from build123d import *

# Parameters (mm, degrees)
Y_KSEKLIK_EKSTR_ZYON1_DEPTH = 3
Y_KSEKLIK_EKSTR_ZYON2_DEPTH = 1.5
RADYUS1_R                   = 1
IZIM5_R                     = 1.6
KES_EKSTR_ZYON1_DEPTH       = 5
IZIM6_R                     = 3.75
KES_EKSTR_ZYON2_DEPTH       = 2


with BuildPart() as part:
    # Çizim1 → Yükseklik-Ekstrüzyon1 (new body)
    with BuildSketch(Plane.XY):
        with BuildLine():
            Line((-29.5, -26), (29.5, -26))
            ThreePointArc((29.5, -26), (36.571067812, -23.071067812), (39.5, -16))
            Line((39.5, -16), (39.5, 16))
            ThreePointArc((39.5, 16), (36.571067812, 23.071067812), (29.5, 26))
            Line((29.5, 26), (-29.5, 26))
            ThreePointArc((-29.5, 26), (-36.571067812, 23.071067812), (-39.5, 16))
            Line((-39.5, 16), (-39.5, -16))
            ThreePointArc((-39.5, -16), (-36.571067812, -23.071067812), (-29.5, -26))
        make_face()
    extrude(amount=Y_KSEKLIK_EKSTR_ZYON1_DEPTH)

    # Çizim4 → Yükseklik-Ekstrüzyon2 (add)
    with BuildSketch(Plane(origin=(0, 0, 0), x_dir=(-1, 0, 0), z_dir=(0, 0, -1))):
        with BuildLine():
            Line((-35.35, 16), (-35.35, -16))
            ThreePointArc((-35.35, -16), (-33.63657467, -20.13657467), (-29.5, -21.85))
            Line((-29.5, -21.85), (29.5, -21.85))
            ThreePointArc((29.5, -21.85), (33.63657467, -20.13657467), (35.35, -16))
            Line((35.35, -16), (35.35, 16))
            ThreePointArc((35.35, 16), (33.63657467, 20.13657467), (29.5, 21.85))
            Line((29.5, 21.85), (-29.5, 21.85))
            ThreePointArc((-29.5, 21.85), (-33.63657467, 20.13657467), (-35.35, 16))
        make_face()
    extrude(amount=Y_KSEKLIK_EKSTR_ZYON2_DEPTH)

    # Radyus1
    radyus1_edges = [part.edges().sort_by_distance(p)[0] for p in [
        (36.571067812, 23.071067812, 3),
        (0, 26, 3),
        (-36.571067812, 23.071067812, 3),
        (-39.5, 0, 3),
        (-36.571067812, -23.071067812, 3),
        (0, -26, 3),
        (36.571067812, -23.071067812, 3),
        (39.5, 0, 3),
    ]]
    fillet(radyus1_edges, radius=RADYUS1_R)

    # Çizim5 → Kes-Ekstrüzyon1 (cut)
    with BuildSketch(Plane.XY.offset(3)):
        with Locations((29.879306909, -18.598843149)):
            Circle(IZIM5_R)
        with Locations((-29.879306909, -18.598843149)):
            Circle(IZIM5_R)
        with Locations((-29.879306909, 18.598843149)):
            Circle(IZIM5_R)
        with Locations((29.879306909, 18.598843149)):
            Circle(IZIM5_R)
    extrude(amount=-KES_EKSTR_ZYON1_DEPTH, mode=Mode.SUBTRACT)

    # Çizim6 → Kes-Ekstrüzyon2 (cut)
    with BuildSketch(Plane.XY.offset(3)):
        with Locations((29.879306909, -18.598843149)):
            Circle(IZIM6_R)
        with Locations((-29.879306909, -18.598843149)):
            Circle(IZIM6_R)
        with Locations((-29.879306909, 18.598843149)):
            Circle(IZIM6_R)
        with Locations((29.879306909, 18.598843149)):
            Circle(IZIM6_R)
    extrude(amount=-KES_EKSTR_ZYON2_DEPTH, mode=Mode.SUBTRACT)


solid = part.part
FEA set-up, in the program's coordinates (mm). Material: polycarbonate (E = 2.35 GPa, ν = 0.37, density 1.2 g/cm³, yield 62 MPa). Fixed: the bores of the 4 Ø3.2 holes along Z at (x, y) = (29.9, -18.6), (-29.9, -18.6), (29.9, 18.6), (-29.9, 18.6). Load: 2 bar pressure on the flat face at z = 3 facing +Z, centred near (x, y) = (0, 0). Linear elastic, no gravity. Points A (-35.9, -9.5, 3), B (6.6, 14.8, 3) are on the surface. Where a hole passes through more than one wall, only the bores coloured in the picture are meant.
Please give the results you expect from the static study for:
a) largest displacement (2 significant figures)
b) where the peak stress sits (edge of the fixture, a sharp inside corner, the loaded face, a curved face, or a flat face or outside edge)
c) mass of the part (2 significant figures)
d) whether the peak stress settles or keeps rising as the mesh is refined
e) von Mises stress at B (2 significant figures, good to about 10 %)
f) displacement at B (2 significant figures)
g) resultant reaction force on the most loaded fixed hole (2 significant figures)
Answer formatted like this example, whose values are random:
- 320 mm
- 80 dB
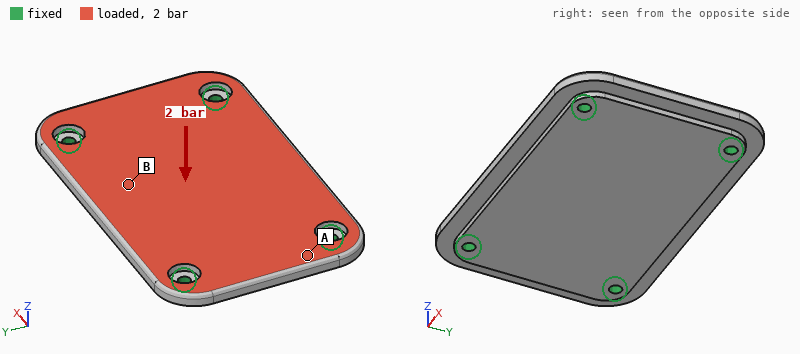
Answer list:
- 0.81 mm
- edge of the fixture
- 19 g
- keeps rising
- 13 MPa
- 0.71 mm
- 260 N
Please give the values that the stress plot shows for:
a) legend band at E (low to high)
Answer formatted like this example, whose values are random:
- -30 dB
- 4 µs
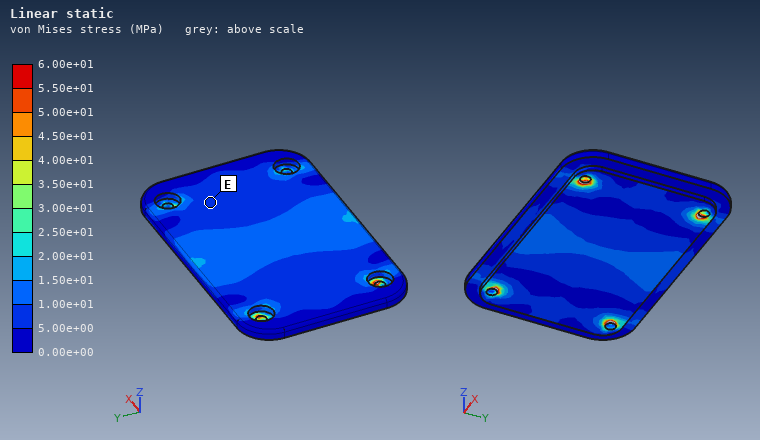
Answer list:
- 5.00e+00 to 1.00e+01 MPa
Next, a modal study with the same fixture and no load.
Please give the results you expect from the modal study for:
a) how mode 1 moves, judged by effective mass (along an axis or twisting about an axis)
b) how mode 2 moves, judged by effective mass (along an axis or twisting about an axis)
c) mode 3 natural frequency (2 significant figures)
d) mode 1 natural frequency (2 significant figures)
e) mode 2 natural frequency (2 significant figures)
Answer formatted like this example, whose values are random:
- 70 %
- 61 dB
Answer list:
- along Z
- twisting about X
- 3000 Hz
- 1200 Hz
- 1800 Hz
